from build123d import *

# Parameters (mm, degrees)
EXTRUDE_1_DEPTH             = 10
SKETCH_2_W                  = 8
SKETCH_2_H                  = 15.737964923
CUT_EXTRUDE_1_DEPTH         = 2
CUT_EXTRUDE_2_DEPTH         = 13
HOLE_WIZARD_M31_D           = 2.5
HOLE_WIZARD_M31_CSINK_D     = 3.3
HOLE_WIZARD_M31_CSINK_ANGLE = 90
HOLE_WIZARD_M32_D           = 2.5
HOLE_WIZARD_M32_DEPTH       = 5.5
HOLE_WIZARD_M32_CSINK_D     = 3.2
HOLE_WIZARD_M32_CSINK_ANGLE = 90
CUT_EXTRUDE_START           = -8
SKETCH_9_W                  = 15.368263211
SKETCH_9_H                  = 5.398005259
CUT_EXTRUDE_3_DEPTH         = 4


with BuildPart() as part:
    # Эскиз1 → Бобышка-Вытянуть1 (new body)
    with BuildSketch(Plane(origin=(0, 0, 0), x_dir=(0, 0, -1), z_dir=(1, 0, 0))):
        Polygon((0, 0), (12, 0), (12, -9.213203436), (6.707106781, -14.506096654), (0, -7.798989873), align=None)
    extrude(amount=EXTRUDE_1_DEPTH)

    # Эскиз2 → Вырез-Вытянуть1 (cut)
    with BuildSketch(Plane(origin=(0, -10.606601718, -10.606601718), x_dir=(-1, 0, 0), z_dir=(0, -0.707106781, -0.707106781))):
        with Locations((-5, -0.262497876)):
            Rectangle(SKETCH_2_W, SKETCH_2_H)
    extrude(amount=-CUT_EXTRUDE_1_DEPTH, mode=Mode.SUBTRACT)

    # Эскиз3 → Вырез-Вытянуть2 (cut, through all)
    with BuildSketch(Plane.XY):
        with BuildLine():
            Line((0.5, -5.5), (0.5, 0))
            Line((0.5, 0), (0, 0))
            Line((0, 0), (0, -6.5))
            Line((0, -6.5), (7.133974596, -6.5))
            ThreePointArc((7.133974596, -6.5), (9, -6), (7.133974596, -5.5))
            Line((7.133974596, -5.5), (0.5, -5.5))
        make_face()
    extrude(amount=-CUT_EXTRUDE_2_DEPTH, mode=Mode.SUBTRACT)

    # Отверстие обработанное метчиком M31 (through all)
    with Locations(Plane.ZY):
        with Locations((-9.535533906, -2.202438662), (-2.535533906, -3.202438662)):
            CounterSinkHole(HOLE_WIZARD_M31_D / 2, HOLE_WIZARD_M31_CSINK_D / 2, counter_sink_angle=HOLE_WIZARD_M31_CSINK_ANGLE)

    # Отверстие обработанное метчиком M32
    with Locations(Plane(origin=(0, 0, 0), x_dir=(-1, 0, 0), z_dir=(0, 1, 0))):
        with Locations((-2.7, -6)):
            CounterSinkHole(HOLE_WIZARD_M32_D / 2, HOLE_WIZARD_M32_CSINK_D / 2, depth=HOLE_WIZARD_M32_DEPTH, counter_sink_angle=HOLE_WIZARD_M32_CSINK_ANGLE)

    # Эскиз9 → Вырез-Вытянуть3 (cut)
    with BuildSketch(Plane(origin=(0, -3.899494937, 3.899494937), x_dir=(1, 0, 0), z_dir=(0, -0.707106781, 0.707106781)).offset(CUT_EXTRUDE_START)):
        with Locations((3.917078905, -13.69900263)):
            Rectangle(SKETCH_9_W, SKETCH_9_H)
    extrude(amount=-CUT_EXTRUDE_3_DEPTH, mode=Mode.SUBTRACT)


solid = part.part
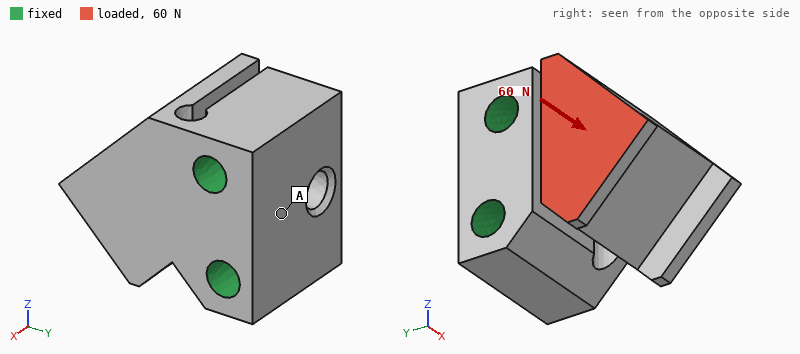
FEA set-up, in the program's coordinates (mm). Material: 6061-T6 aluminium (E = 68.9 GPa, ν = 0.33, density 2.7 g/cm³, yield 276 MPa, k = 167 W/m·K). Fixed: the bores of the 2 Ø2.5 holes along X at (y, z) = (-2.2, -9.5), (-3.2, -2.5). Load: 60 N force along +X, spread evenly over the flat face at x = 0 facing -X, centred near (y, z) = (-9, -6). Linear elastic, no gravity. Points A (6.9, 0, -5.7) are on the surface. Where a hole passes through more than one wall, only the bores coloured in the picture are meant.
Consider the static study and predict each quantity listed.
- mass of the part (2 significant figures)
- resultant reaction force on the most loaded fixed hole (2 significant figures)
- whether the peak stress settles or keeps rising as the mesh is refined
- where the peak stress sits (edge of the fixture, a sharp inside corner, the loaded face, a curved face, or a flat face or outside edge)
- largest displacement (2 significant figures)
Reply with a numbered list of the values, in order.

1. 2.5 g
2. 31 N
3. keeps rising
4. a sharp inside corner
5. 86 µm
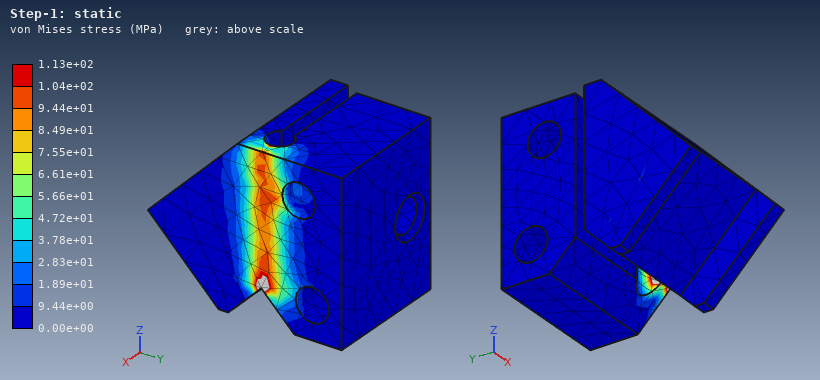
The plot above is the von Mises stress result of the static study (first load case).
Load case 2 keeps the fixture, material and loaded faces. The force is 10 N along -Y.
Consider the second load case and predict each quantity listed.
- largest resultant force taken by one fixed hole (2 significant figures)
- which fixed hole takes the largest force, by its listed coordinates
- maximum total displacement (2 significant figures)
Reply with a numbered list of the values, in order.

1. 6.1 N
2. (-2.2, -9.5)
3. 39 µm
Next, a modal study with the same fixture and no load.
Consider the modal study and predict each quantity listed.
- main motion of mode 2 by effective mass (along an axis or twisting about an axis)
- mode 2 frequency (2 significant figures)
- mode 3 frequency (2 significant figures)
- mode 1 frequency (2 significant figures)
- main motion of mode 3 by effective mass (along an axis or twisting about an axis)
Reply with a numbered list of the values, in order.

1. along Z
2. 12 kHz
3. 28 kHz
4. 4000 Hz
5. along X
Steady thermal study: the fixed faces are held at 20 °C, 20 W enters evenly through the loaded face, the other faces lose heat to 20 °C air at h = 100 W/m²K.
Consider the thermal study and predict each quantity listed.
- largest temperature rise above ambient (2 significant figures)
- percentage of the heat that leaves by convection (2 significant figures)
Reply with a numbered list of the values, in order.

1. 67 K
2. 8.7 %
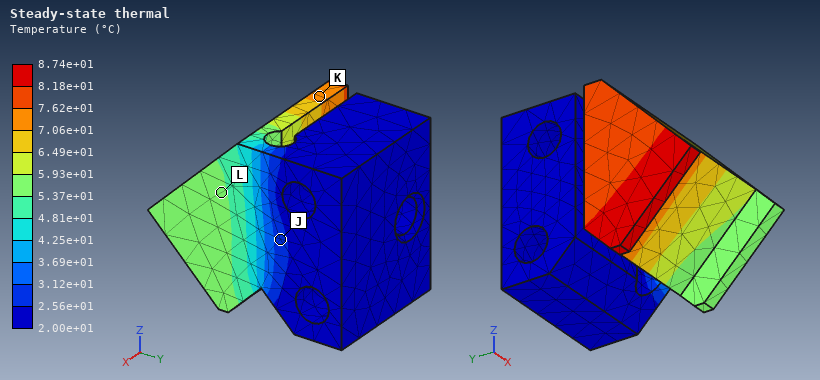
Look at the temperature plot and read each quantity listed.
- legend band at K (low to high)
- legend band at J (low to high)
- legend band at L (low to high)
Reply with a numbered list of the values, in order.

1. 7.06e+01 to 7.62e+01 °C
2. 2.56e+01 to 3.12e+01 °C
3. 5.37e+01 to 5.93e+01 °C
